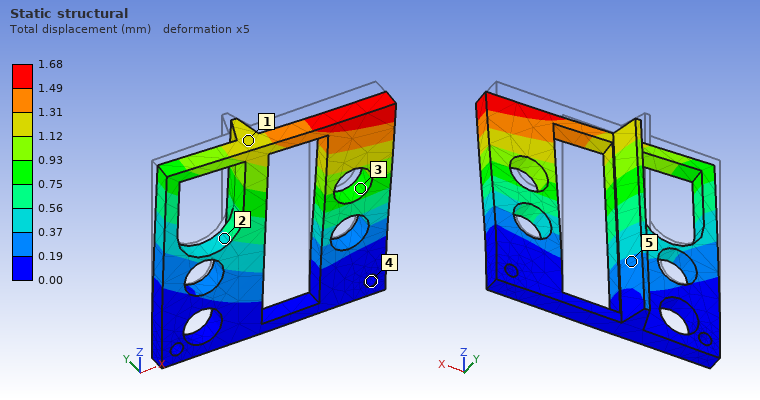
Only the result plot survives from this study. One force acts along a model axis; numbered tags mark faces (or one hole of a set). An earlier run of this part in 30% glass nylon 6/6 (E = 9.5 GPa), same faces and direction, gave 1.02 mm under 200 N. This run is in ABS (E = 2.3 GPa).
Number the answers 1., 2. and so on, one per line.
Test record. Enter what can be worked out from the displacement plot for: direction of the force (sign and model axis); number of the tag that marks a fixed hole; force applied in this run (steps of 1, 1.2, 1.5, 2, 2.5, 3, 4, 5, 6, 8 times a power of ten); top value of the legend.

1. -Y
2. 4
3. 80 N
4. 1.68 mm
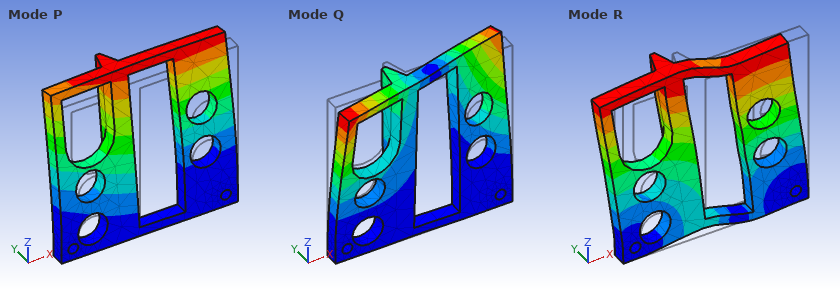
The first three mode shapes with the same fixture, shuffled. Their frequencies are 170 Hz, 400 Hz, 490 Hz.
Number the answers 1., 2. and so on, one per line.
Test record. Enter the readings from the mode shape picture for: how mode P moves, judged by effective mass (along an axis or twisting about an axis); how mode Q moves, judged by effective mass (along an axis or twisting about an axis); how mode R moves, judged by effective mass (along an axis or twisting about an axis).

1. along Y
2. twisting about Z
3. along X
